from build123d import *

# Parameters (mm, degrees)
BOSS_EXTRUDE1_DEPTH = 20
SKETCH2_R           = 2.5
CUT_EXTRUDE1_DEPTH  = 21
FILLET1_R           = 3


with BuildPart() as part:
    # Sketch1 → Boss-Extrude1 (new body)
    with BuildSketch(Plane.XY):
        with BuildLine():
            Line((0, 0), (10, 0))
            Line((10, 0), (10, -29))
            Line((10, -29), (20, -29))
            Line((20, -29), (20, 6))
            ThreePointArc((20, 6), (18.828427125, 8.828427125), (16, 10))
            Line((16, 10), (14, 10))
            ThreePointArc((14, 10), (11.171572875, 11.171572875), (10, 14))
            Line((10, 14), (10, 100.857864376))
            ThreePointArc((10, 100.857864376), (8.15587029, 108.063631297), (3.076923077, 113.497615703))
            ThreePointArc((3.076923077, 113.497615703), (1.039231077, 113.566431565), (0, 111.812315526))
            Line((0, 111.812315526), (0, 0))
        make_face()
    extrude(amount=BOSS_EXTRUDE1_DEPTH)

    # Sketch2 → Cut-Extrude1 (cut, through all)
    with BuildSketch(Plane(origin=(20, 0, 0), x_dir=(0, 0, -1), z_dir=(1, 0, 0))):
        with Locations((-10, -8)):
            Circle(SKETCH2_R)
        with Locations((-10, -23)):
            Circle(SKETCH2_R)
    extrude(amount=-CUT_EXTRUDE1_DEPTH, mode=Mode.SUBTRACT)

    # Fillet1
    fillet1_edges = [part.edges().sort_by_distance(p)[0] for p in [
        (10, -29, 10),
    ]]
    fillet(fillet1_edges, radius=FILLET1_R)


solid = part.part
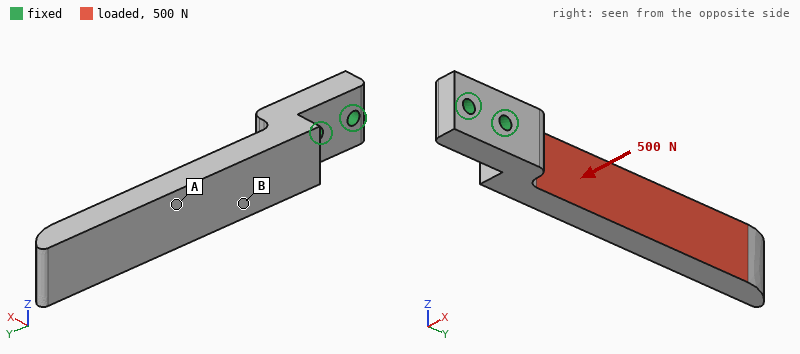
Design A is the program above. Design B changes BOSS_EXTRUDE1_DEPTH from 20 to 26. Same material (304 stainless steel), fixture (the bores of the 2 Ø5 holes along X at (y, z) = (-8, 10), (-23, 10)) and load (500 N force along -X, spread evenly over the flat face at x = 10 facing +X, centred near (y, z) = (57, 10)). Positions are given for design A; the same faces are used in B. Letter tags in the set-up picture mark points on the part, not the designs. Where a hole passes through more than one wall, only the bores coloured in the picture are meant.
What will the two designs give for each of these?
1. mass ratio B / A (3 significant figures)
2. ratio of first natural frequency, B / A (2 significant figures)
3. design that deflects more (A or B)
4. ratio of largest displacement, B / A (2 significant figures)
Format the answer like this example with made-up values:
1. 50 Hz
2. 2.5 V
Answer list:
1. 1.30
2. 0.99
3. A
4. 0.79
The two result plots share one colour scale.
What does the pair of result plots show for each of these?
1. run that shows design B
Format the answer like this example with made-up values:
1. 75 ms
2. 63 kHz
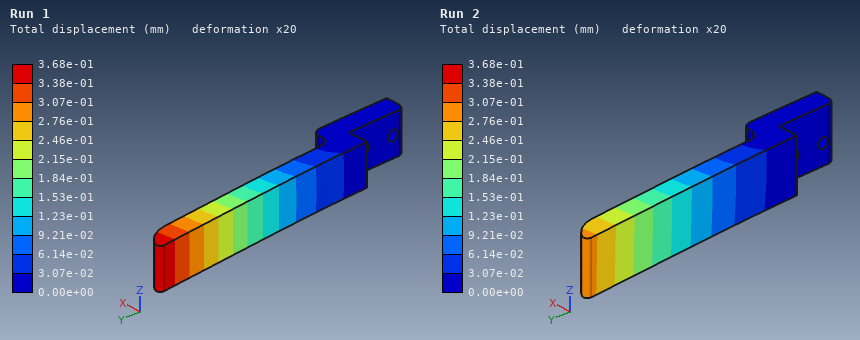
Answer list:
1. Run 2
